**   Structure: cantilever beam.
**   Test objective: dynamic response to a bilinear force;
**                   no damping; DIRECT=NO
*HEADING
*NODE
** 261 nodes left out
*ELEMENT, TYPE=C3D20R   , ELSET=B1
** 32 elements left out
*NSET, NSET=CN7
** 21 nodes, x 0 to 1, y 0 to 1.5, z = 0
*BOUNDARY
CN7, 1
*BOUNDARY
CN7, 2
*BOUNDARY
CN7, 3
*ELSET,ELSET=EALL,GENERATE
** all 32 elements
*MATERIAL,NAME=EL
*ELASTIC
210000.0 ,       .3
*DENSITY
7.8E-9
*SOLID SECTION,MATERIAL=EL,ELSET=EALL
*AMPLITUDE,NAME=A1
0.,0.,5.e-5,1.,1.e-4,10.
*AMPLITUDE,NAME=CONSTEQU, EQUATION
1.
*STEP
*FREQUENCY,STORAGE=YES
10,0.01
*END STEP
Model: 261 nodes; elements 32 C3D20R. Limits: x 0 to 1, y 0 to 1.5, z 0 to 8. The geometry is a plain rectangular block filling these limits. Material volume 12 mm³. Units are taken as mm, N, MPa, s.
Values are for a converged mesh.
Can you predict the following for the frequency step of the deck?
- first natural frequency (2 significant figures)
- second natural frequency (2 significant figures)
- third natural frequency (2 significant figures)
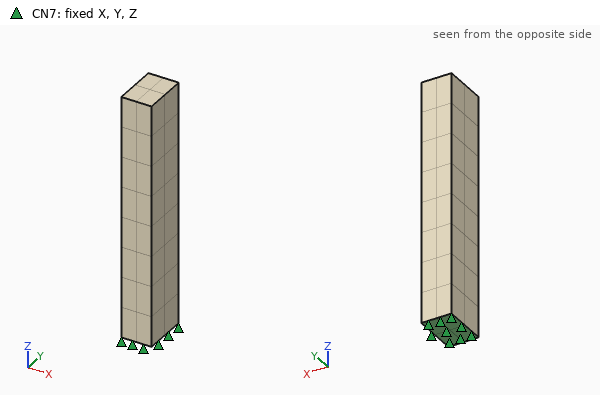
13000 Hz
19000 Hz
77000 Hz
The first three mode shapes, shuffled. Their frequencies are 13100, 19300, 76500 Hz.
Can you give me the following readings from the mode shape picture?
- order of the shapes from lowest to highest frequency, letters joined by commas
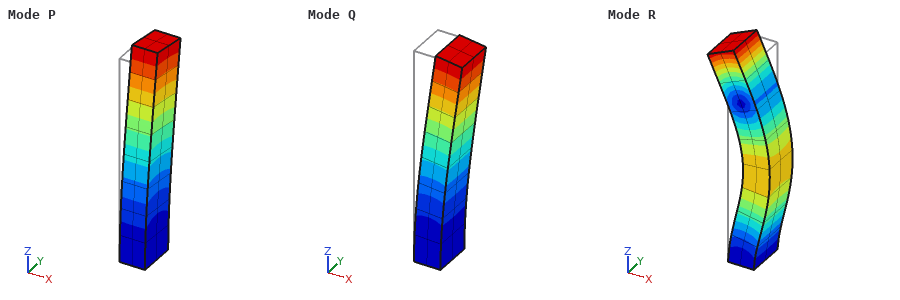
Q, P, R
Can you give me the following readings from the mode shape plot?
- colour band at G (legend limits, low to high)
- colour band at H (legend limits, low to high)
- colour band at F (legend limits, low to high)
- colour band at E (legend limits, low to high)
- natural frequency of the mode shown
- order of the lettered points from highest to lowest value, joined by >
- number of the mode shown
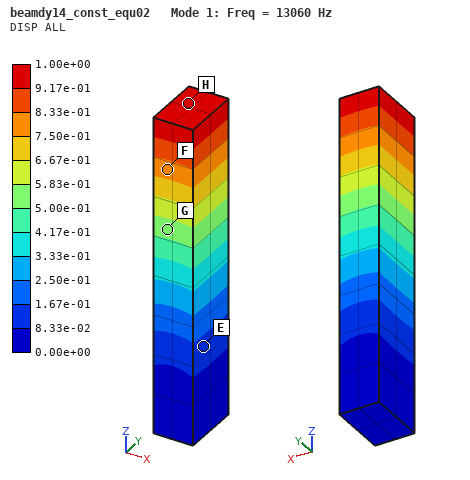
5.00e-01 to 5.83e-01
9.17e-01 to 1.00e+00
7.50e-01 to 8.33e-01
8.33e-02 to 1.67e-01
13060 Hz
H > F > G > E
1
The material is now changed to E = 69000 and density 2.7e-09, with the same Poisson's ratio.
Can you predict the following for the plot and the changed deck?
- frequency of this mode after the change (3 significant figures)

12700 Hz
